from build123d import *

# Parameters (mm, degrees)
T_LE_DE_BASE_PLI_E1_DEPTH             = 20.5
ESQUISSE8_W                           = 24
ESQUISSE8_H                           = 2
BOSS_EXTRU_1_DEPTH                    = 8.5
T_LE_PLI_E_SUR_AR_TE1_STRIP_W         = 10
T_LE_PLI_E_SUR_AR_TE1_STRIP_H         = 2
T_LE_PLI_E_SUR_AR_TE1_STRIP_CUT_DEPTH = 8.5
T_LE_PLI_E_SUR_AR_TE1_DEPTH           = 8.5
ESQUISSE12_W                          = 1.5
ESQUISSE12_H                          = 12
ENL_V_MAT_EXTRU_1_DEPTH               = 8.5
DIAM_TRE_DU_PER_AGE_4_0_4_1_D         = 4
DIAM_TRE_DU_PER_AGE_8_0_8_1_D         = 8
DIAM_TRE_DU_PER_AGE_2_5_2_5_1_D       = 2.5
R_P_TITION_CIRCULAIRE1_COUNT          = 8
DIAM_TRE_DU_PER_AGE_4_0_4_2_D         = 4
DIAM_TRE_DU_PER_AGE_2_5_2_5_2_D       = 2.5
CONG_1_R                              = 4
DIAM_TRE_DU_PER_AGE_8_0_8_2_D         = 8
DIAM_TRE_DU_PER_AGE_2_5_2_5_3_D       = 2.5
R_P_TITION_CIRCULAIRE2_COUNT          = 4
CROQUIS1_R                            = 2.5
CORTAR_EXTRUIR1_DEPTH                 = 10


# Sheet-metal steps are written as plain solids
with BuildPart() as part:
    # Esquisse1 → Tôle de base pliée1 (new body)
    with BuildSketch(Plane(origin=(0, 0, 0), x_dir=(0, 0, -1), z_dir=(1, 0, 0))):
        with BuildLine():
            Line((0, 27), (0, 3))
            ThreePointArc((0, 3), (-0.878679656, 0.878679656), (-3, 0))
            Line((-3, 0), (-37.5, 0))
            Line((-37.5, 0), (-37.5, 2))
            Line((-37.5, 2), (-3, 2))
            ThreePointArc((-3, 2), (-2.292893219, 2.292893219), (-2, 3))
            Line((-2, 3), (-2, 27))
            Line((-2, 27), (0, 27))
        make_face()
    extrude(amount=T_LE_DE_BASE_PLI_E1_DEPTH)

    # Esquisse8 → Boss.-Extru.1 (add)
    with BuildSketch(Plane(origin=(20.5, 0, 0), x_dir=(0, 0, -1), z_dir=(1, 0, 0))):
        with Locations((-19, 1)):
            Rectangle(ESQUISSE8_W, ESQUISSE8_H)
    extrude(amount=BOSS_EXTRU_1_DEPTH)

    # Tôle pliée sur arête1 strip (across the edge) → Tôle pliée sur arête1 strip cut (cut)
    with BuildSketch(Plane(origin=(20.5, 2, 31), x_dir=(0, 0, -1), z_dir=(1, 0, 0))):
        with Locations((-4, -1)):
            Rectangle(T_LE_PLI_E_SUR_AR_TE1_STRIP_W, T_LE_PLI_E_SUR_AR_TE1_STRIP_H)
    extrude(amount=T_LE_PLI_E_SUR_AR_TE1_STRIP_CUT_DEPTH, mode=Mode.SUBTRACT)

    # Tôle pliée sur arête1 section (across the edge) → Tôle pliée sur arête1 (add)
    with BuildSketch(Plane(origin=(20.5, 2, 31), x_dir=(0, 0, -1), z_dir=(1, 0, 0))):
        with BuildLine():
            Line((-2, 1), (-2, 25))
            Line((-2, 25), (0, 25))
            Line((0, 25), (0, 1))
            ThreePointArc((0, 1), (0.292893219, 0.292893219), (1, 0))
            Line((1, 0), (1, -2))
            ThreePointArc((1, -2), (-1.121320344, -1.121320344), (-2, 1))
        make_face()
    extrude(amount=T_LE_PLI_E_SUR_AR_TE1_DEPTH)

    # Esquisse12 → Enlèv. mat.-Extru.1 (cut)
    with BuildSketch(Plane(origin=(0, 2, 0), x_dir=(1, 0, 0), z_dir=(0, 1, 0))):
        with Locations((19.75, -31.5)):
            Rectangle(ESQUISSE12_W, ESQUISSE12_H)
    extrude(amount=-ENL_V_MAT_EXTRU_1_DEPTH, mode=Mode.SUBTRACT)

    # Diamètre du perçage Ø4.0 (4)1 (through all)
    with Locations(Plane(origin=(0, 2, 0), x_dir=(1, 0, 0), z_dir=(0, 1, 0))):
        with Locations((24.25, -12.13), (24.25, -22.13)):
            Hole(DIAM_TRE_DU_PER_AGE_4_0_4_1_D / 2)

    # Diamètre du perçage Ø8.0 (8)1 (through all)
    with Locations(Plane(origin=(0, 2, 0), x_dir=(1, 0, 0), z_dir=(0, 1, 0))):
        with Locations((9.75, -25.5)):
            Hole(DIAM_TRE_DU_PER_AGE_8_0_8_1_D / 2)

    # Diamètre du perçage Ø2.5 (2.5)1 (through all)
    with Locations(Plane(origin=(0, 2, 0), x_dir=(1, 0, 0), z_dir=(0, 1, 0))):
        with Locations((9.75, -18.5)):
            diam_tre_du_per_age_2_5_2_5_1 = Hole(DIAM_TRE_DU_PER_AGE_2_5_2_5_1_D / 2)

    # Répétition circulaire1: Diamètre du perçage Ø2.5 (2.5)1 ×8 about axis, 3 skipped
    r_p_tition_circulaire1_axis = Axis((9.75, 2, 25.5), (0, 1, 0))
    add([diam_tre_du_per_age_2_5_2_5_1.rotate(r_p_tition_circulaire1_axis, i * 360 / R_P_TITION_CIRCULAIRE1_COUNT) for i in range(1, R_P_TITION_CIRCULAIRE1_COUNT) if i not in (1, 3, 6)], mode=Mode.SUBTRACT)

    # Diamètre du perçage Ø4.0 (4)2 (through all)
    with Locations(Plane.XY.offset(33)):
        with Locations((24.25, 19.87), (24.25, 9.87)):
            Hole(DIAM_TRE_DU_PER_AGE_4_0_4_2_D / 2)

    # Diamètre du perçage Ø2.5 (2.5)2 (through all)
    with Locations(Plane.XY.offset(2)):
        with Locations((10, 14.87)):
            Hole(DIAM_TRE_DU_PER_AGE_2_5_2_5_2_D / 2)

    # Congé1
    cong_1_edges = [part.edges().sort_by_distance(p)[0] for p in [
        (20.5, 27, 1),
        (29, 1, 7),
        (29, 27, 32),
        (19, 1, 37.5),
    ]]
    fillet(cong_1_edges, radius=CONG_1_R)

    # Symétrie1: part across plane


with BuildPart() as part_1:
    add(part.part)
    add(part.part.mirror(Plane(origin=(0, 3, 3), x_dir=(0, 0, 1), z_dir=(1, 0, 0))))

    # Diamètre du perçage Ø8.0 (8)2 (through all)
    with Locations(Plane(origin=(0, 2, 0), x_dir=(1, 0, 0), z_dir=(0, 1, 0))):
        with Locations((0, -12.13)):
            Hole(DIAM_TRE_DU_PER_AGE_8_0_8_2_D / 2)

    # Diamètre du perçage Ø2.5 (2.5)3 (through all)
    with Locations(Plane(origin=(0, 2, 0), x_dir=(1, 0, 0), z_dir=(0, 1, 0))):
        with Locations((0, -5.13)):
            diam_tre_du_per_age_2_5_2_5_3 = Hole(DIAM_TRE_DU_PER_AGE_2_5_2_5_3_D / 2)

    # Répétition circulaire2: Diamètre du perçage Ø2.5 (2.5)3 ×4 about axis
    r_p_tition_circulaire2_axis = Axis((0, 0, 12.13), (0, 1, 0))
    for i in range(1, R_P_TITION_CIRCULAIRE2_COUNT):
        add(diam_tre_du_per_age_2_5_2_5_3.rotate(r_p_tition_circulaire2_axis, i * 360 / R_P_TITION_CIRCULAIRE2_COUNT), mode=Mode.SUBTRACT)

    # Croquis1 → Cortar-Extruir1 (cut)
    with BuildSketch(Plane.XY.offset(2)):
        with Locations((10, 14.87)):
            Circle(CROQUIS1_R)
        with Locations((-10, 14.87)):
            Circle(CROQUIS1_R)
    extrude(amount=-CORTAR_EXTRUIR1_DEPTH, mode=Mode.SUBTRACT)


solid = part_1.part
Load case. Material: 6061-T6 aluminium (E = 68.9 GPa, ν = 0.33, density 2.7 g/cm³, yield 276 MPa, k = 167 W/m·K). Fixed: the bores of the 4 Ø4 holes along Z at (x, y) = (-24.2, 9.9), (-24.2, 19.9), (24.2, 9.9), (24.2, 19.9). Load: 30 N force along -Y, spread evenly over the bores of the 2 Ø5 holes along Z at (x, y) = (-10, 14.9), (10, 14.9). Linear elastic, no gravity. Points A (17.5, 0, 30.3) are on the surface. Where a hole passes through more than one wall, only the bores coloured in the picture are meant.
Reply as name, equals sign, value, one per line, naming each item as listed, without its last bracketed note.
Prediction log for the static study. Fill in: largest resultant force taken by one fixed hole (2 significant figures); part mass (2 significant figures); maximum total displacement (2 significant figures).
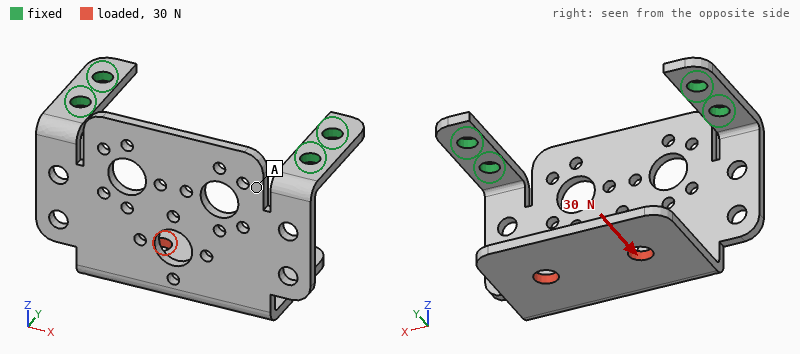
largest resultant force taken by one fixed hole = 15 N
part mass = 16 g
maximum total displacement = 0.83 mm
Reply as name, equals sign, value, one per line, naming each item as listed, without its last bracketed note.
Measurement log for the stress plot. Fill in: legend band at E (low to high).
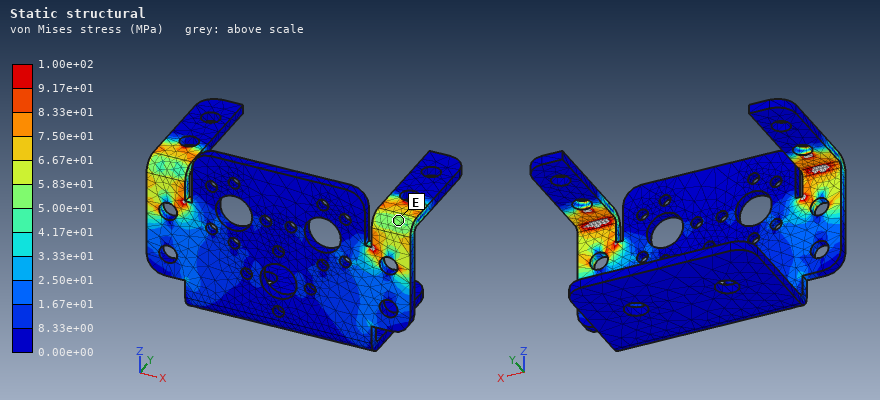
legend band at E = 5.00e+01 to 5.83e+01 MPa
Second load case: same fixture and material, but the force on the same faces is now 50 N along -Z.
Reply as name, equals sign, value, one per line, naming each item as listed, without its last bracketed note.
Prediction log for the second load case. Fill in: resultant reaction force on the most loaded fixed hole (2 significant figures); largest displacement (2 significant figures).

resultant reaction force on the most loaded fixed hole = 26 N
largest displacement = 0.79 mm
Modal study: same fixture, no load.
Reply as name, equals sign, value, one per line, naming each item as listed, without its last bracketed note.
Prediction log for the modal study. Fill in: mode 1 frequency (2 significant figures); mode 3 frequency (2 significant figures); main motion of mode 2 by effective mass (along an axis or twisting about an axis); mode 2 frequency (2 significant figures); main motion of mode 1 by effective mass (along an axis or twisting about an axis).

mode 1 frequency = 380 Hz
mode 3 frequency = 1400 Hz
main motion of mode 2 by effective mass = along X
mode 2 frequency = 1100 Hz
main motion of mode 1 by effective mass = along Y
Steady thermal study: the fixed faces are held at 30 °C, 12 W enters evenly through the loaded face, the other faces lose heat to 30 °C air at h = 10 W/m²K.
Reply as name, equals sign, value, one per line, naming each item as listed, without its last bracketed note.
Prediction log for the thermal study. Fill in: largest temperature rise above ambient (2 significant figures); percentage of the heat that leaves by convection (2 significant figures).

largest temperature rise above ambient = 64 K
percentage of the heat that leaves by convection = 23 %
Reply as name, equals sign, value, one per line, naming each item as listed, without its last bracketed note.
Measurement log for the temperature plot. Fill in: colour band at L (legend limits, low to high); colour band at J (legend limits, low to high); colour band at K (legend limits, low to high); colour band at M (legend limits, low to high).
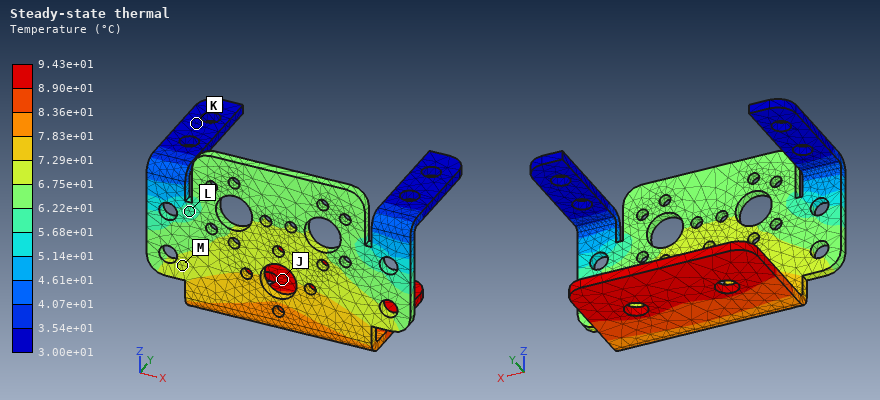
colour band at L = 5.68e+01 to 6.22e+01 °C
colour band at J = 8.90e+01 to 9.43e+01 °C
colour band at K = 3.00e+01 to 3.54e+01 °C
colour band at M = 6.75e+01 to 7.29e+01 °C
